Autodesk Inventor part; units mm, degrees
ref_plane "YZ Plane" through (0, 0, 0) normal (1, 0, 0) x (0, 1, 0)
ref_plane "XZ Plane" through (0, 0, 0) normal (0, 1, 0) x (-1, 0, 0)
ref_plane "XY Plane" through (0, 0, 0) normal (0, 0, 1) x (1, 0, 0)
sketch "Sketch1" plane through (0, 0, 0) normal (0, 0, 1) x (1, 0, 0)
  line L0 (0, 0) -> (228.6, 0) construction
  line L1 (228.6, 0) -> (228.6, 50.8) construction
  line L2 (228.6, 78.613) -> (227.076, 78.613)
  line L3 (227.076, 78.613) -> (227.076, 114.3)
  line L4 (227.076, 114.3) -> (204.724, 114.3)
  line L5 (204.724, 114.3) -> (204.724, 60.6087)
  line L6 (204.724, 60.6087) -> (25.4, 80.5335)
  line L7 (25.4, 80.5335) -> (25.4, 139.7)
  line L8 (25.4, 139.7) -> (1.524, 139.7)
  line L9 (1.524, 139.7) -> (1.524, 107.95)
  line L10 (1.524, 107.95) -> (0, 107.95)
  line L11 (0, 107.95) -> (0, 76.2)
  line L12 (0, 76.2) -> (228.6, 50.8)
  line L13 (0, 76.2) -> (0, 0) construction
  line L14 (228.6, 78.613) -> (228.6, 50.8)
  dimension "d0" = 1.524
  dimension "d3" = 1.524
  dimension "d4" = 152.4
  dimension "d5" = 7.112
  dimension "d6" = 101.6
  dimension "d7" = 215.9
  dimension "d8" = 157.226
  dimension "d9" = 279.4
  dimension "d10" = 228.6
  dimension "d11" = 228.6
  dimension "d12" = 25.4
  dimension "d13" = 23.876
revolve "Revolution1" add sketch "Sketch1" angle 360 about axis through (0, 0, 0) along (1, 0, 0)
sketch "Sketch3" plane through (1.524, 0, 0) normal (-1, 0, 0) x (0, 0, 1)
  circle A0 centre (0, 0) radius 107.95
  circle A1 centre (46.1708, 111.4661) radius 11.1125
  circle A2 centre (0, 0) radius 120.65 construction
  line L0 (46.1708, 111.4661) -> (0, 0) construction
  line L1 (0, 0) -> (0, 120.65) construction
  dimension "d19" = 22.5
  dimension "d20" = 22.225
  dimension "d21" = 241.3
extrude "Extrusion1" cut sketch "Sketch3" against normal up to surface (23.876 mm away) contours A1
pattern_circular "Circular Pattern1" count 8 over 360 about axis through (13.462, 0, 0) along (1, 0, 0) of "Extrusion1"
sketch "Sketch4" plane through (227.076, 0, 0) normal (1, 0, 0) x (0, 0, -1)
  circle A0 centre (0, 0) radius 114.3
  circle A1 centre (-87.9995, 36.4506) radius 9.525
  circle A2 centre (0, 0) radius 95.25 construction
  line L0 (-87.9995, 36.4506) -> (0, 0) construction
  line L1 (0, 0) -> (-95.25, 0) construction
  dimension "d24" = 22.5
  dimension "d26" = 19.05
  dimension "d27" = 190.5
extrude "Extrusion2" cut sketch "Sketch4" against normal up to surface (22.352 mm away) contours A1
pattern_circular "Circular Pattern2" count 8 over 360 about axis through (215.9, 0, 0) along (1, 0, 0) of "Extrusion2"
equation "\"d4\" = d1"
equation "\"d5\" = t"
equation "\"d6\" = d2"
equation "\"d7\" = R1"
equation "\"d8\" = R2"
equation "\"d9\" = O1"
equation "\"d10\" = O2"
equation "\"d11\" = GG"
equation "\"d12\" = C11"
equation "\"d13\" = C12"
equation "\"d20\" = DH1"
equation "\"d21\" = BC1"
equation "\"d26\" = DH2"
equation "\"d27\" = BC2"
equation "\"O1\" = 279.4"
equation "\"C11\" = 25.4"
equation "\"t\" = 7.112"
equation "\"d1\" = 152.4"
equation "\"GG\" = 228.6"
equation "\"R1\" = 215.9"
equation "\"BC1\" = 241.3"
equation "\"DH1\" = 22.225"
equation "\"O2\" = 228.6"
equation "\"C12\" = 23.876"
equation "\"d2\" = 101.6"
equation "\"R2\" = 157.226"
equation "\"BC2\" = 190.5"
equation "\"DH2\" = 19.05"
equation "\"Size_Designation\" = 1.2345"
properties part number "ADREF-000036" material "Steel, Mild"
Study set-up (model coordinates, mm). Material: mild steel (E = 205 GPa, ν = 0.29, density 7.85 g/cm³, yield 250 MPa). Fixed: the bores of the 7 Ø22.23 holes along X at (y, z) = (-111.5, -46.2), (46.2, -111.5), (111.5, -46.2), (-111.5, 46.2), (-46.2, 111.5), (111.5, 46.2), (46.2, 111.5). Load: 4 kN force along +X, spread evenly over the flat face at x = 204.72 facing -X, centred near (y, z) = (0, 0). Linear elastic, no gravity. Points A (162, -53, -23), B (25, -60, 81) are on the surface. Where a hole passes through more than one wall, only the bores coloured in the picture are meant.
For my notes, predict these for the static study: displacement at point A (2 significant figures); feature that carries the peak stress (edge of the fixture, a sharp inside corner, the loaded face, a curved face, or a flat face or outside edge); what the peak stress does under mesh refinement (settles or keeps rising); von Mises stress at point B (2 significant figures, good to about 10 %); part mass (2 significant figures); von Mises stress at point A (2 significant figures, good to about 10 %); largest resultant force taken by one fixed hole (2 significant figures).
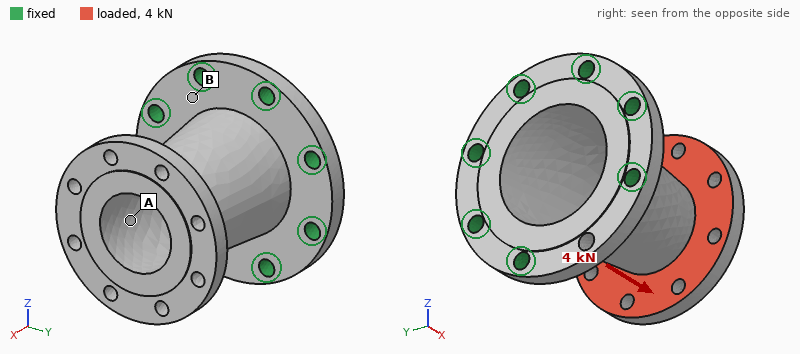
1.8 µm
edge of the fixture
keeps rising
0.75 MPa
18 kg
2.1 MPa
770 N
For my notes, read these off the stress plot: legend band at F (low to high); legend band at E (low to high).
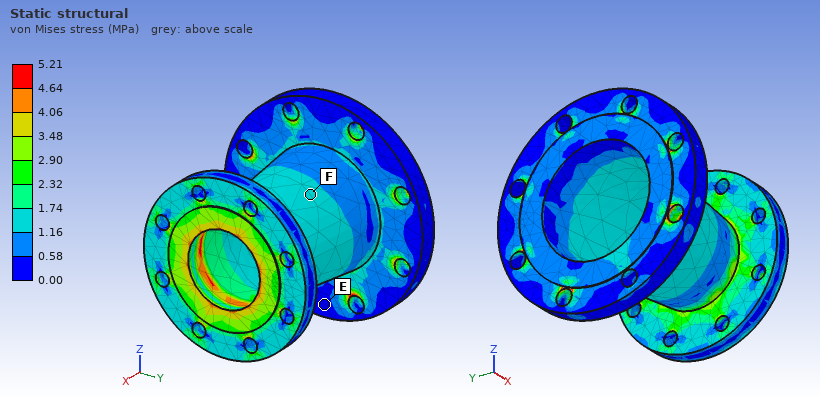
1.16 to 1.74 MPa
0.00 to 0.58 MPa
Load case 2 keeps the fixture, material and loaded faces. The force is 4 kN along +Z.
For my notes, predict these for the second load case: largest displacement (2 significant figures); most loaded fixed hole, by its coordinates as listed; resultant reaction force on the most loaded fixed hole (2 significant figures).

20 µm
(46.2, -111.5)
3.1 kN
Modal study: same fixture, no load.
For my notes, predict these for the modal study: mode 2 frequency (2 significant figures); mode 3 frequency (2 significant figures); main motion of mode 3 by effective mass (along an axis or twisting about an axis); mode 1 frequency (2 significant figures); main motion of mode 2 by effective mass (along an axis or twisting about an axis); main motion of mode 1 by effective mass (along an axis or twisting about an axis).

930 Hz
1700 Hz
twisting about X
870 Hz
along Y
along Z
